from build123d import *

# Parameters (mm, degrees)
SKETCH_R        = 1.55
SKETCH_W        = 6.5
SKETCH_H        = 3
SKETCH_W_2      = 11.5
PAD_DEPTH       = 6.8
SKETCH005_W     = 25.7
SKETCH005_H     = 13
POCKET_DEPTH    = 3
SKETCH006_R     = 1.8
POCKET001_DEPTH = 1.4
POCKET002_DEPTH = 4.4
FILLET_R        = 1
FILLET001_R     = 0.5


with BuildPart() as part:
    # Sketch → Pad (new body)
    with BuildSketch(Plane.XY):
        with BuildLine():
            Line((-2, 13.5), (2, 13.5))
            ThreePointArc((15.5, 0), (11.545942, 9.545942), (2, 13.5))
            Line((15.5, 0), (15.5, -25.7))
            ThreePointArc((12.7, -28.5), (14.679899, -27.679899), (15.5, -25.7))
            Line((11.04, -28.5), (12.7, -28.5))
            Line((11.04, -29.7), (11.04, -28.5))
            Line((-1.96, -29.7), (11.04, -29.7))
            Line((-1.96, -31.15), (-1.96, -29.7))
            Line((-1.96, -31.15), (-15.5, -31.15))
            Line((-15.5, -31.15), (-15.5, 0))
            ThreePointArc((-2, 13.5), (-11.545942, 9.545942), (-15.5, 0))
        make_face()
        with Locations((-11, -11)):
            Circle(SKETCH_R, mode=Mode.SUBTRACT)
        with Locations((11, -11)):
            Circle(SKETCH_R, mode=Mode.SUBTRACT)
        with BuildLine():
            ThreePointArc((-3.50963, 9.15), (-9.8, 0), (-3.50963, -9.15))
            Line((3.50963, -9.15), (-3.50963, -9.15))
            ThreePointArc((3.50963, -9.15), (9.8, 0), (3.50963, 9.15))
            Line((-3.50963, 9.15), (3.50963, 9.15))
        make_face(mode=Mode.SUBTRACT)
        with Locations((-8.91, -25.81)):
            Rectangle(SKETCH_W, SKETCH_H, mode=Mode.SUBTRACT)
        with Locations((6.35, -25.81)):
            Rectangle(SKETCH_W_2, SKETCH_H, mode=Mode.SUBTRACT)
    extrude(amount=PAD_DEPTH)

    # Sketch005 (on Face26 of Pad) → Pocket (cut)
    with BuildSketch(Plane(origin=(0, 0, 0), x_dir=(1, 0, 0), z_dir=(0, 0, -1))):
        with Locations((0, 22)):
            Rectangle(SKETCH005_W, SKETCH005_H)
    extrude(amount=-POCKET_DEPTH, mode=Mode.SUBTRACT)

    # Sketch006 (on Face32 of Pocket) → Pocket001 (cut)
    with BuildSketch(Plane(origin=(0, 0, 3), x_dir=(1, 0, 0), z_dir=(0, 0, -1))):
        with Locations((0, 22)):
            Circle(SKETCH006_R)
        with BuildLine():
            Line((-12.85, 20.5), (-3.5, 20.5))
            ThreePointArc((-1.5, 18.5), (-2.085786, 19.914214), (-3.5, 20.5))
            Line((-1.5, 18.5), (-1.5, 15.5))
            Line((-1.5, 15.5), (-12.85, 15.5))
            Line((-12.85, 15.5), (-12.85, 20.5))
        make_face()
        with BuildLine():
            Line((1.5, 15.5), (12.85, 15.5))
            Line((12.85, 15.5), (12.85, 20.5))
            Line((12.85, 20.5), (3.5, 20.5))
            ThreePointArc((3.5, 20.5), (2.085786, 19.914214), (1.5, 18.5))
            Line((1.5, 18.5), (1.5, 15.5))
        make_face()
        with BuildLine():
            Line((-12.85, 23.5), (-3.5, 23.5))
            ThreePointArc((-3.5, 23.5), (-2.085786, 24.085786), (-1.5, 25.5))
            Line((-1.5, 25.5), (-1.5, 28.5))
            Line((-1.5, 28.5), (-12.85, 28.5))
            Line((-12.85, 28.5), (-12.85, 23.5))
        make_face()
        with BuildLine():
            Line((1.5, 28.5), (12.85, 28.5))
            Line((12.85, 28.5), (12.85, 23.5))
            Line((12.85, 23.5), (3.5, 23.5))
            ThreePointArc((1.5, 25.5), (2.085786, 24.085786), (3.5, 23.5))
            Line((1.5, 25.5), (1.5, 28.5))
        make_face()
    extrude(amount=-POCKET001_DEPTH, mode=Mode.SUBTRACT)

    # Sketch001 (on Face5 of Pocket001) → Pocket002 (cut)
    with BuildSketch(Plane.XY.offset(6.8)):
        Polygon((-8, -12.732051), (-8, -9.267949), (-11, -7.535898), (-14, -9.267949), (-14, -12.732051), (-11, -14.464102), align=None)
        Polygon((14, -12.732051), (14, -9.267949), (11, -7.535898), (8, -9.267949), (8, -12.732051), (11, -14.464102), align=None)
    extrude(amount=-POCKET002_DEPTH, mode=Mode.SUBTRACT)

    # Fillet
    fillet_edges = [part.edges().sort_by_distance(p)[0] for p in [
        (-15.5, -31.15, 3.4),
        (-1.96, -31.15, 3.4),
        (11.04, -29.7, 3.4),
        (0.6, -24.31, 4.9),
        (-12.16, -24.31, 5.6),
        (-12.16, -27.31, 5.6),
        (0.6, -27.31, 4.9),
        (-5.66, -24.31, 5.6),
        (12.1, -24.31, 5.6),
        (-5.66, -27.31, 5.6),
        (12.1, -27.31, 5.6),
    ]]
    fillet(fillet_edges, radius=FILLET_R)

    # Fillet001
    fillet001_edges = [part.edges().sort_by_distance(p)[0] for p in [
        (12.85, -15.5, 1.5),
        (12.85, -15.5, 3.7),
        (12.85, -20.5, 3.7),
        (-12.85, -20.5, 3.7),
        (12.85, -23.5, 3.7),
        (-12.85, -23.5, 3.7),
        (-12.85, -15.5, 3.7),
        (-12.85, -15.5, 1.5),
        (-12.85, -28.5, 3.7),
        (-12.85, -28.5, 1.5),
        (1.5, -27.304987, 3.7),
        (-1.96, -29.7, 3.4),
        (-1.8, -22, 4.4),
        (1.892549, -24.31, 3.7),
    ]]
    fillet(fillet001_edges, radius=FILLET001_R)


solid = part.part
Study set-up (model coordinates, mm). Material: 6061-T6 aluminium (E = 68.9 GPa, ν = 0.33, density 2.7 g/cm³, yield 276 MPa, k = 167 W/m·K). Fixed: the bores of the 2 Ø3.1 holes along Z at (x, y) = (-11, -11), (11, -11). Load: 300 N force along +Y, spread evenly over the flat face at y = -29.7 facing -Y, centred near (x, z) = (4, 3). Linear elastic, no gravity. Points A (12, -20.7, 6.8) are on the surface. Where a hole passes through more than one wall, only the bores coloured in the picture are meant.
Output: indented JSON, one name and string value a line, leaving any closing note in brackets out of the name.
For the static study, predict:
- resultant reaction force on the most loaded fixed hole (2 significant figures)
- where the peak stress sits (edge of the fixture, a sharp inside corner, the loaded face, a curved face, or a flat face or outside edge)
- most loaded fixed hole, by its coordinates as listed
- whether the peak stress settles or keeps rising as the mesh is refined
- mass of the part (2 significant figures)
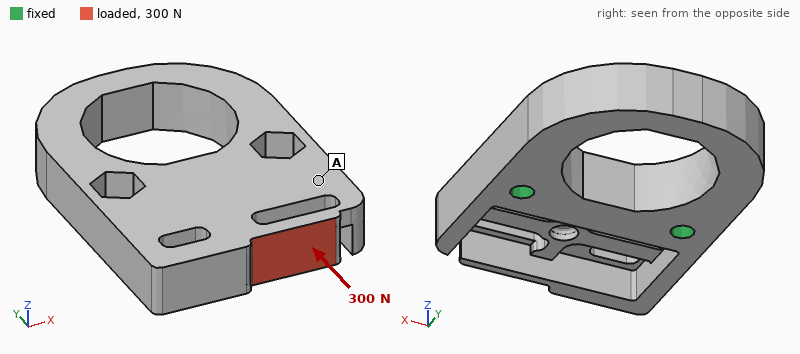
{
  "resultant reaction force on the most loaded fixed hole": "200 N",
  "where the peak stress sits": "a sharp inside corner",
  "most loaded fixed hole, by its coordinates as listed": "(11, -11)",
  "whether the peak stress settles or keeps rising as the mesh is refined": "keeps rising",
  "mass of the part": "13 g"
}
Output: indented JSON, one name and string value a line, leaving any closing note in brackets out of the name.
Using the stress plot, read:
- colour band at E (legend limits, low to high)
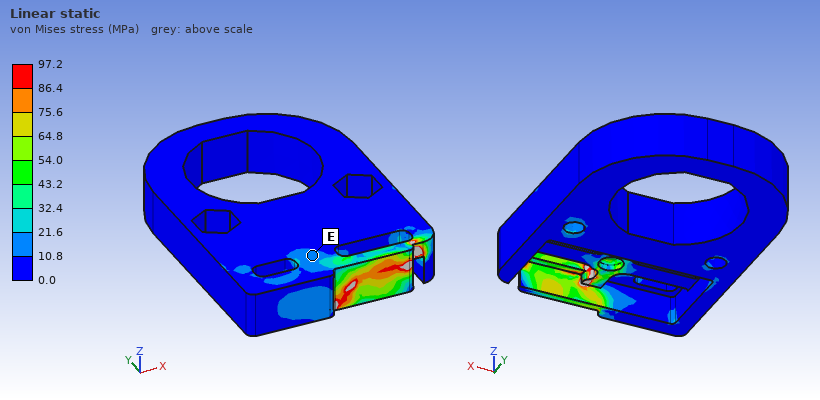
{
  "colour band at E": "10.8 to 21.6 MPa"
}
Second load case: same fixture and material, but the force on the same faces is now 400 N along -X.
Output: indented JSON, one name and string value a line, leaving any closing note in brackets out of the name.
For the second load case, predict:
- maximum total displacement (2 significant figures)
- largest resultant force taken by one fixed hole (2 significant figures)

{
  "maximum total displacement": "33 µm",
  "largest resultant force taken by one fixed hole": "370 N"
}
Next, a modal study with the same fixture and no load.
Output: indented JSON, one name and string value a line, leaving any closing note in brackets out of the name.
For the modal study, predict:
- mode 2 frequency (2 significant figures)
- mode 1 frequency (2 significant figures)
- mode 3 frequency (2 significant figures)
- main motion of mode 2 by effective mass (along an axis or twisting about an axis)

{
  "mode 2 frequency": "8300 Hz",
  "mode 1 frequency": "4500 Hz",
  "mode 3 frequency": "10 kHz",
  "main motion of mode 2 by effective mass": "along Z"
}
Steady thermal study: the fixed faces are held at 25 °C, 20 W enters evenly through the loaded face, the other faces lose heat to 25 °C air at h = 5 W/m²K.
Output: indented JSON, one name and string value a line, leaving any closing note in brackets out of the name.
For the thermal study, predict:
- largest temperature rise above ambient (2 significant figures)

{
  "largest temperature rise above ambient": "71 K"
}
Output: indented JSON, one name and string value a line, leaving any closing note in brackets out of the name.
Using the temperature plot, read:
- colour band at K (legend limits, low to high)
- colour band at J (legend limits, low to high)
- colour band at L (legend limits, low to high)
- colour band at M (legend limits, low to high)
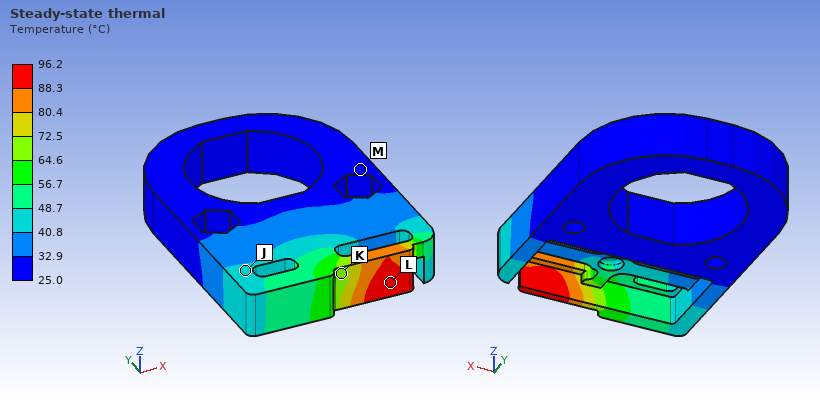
{
  "colour band at K": "64.6 to 72.5 °C",
  "colour band at J": "40.8 to 48.7 °C",
  "colour band at L": "88.3 to 96.2 °C",
  "colour band at M": "25.0 to 32.9 °C"
}
